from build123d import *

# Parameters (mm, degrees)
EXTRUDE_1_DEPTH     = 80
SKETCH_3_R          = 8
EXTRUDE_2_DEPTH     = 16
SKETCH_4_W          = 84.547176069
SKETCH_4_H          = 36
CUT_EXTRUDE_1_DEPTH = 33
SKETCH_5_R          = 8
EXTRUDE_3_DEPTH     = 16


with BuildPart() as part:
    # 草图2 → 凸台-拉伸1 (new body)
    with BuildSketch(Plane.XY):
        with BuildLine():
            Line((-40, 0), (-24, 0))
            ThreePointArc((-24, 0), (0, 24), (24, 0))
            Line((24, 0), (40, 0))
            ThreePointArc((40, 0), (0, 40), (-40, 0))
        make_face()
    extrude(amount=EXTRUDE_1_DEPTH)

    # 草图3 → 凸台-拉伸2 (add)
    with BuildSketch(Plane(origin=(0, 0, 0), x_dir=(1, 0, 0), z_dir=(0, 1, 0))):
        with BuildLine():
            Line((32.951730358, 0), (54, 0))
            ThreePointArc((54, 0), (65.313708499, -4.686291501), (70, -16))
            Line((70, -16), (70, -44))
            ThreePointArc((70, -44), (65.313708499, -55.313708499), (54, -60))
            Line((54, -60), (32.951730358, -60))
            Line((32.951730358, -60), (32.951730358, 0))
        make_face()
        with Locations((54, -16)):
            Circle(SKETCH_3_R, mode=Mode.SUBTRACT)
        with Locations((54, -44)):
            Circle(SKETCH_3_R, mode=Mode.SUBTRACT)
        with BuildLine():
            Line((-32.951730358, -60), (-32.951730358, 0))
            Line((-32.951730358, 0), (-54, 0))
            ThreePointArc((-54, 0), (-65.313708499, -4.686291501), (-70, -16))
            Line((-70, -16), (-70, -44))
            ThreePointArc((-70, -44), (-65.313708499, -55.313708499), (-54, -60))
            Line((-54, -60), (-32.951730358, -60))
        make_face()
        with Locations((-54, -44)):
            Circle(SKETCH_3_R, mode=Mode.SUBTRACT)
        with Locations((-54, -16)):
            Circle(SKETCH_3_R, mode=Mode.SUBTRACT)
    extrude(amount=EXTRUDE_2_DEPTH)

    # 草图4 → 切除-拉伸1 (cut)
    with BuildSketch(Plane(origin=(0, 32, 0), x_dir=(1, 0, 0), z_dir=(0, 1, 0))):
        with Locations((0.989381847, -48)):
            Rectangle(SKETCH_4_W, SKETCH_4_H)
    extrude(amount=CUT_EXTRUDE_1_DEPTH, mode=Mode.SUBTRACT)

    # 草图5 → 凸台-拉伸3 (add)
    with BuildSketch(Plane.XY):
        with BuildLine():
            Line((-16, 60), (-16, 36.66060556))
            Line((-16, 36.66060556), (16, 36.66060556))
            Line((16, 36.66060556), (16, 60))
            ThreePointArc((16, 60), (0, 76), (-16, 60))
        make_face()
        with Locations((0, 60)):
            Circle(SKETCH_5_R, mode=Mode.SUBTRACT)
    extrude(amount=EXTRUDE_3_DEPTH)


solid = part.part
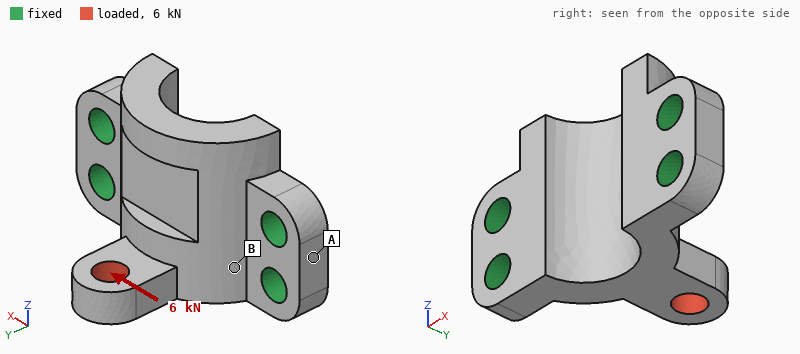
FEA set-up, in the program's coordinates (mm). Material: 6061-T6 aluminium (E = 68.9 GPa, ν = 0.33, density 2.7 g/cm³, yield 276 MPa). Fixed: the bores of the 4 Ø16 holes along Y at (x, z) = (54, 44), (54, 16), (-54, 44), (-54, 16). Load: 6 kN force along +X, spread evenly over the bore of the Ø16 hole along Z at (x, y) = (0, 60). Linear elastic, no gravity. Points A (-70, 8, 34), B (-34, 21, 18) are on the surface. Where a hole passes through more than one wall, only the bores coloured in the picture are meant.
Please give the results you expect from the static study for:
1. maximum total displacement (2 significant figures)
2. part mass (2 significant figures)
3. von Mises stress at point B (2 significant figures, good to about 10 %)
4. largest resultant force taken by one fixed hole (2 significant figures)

96 µm
480 g
17 MPa
3.3 kN
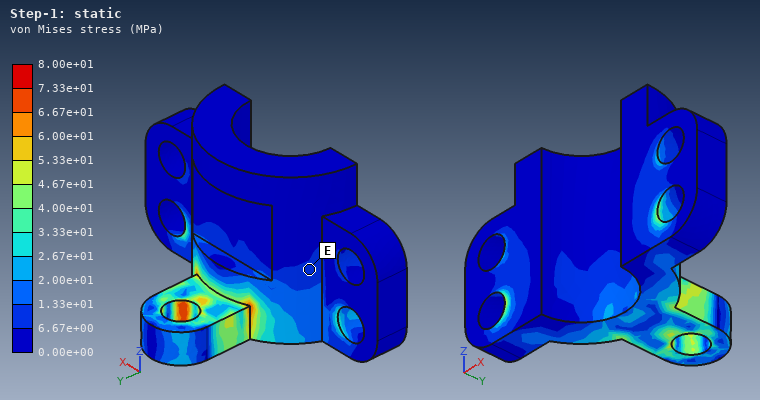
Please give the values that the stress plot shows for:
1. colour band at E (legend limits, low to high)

6.67e+00 to 1.33e+01 MPa
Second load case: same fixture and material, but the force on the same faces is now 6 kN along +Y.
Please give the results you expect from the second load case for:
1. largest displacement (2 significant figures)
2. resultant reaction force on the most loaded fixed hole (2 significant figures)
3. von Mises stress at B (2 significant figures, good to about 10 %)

49 µm
4.2 kN
12 MPa
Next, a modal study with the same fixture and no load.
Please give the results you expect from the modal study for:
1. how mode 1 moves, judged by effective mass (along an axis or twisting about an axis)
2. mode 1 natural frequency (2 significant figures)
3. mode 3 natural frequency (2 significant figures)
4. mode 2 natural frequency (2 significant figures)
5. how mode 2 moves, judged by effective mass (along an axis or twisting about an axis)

along Z
4600 Hz
8100 Hz
7300 Hz
along Y
